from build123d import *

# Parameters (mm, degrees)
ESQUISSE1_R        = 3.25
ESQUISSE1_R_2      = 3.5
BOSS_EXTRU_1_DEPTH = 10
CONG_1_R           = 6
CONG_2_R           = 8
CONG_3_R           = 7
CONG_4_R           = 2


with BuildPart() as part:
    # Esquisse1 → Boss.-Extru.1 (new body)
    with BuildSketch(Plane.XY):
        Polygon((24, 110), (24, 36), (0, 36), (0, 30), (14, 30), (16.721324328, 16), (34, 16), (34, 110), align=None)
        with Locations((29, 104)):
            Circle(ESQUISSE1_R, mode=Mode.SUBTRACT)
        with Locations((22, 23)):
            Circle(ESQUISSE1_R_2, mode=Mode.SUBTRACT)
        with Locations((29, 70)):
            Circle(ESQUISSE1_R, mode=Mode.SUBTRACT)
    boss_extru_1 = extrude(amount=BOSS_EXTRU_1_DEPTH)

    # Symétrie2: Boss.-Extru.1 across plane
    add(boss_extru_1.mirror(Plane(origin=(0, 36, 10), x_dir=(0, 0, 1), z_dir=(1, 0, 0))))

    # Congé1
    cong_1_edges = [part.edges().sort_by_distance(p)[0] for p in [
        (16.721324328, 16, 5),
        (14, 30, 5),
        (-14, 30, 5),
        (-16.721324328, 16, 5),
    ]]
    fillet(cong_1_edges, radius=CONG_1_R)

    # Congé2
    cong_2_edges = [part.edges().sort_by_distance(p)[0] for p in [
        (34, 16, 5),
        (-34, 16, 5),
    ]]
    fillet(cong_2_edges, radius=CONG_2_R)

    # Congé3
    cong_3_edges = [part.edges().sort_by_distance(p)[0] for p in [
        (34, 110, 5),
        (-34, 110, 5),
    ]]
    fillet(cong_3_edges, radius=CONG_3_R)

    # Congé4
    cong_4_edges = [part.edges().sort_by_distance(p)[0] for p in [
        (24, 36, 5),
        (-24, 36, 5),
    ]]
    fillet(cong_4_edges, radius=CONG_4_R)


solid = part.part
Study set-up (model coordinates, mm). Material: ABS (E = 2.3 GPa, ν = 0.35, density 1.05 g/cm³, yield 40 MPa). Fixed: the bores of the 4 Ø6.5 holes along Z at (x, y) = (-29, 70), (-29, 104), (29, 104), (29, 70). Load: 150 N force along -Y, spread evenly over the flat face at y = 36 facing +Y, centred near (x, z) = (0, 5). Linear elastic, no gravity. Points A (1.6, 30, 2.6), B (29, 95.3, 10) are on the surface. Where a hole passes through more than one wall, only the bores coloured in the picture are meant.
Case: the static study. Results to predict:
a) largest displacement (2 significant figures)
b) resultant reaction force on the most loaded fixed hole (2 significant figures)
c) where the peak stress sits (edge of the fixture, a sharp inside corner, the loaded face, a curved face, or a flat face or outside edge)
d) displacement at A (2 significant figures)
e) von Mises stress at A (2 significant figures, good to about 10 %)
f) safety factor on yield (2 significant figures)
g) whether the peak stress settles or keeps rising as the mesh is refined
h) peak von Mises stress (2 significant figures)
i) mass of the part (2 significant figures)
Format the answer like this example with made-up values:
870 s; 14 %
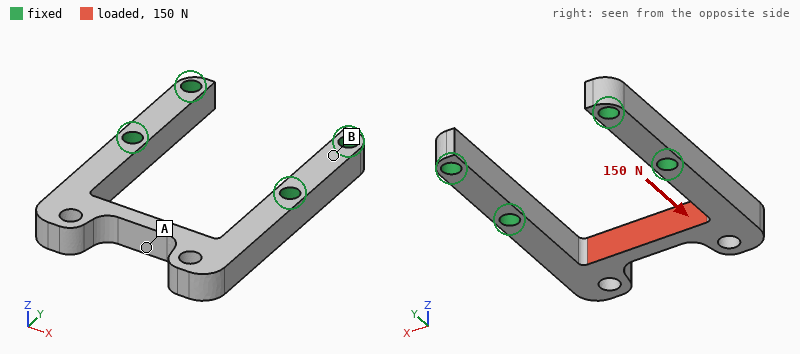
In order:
0.19 mm; 85 N; a curved face; 0.18 mm; 6.2 MPa; 3.5; settles; 11 MPa; 23 g
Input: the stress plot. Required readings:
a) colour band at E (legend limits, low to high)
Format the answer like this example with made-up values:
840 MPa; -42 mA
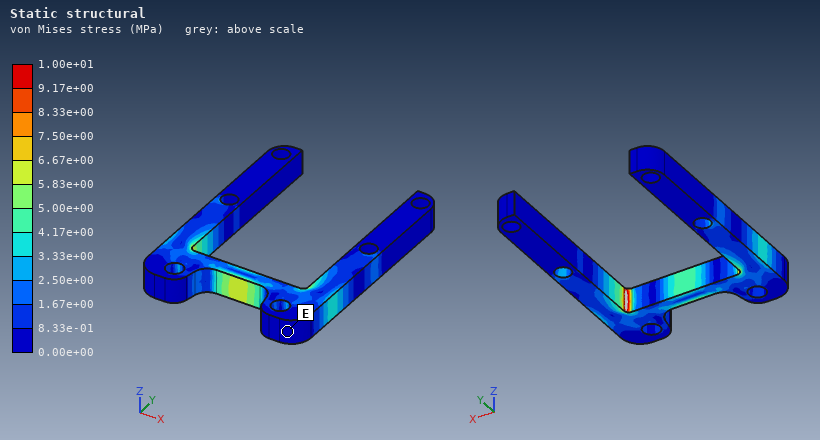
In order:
0.00e+00 to 8.33e-01 MPa
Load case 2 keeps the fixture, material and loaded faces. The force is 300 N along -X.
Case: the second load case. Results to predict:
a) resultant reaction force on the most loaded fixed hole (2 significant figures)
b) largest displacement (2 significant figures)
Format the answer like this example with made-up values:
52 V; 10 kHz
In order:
160 N; 0.76 mm
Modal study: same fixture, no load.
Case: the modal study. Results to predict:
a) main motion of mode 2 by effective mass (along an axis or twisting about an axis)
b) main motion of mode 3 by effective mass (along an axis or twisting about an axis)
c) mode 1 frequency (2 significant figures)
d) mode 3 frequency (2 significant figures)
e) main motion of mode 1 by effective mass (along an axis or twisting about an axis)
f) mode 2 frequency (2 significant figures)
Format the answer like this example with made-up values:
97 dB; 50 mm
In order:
twisting about Y; along X; 670 Hz; 1000 Hz; along Z; 990 Hz
